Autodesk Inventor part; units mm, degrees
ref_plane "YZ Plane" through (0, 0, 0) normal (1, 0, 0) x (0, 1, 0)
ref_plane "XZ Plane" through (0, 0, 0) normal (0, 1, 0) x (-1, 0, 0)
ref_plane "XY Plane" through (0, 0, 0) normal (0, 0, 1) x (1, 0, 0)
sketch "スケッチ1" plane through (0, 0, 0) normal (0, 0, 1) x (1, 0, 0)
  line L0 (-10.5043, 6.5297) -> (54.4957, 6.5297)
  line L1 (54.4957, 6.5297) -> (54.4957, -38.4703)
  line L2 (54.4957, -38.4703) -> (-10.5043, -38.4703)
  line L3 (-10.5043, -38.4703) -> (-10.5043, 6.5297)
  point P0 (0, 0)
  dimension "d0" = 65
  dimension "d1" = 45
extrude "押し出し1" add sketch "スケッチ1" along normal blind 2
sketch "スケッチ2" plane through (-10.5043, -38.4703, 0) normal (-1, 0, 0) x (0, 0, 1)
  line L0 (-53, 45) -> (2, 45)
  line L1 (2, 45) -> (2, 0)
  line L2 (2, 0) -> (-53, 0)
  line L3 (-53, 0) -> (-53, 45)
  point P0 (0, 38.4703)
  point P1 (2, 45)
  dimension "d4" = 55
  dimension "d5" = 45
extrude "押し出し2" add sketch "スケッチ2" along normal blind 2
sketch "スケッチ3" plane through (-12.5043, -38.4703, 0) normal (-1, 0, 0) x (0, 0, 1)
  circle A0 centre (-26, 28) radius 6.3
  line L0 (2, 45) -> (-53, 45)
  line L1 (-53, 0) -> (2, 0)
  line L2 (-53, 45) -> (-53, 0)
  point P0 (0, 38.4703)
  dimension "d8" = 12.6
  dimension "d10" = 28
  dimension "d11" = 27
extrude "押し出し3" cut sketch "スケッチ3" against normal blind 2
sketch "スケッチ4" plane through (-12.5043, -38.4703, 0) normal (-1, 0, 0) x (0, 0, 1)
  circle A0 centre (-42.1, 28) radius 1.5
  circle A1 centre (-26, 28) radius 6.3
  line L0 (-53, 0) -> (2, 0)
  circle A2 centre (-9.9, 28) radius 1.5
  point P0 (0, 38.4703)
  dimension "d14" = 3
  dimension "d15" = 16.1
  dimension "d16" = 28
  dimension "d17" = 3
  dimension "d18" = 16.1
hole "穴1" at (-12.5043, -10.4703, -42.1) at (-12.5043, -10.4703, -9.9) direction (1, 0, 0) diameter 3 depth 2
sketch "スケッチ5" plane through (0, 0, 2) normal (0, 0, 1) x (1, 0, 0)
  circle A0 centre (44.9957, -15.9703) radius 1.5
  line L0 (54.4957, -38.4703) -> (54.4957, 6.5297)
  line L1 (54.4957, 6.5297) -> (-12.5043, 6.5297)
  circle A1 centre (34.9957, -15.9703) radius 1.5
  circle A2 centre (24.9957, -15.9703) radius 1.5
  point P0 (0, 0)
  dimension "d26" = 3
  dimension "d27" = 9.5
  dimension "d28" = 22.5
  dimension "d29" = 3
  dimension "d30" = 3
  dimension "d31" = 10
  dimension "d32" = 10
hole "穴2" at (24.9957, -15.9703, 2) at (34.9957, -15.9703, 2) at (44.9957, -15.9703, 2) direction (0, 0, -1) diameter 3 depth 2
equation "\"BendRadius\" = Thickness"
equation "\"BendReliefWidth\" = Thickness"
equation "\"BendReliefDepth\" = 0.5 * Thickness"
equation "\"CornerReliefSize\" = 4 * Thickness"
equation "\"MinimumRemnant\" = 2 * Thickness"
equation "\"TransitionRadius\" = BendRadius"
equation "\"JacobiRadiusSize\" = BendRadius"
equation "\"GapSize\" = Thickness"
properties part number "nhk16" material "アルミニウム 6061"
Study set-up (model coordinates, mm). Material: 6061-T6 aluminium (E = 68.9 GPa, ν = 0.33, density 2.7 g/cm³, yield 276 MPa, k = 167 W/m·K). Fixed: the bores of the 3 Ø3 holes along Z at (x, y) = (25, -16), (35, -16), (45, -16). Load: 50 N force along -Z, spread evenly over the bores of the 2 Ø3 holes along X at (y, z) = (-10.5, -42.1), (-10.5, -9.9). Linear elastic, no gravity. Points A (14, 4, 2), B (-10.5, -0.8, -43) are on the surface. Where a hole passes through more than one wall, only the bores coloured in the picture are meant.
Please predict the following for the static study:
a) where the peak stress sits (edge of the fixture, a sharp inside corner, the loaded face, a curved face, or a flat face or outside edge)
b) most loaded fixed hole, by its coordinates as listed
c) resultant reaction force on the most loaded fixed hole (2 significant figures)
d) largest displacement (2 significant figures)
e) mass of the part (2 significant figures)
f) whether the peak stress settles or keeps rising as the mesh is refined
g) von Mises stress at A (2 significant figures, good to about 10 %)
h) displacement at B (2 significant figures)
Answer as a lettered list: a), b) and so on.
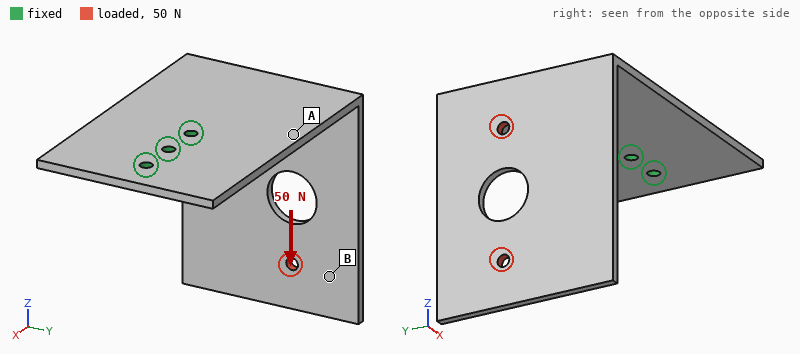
a) edge of the fixture
b) (25, -16)
c) 130 N
d) 1.1 mm
e) 28 g
f) keeps rising
g) 39 MPa
h) 0.90 mm
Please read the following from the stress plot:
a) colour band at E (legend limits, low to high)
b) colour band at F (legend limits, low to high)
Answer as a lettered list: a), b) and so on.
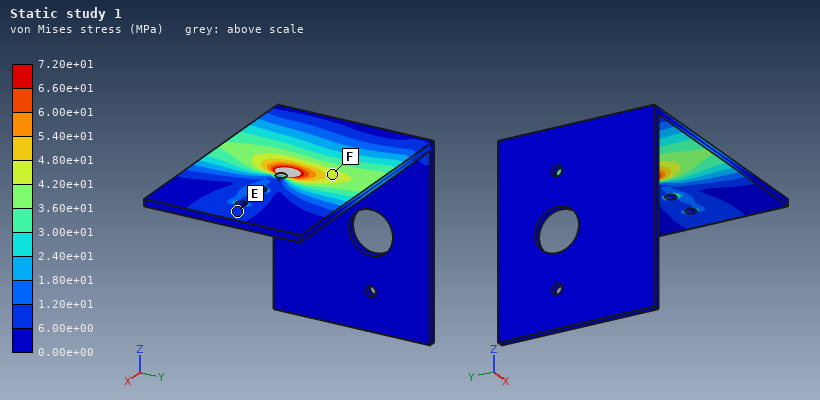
a) 6.00e+00 to 1.20e+01 MPa
b) 4.20e+01 to 4.80e+01 MPa
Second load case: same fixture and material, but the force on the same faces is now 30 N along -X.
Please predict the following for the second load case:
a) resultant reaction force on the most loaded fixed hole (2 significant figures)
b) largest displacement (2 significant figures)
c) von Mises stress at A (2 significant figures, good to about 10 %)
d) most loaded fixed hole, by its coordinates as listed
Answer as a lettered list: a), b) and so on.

a) 44 N
b) 1.1 mm
c) 25 MPa
d) (25, -16)
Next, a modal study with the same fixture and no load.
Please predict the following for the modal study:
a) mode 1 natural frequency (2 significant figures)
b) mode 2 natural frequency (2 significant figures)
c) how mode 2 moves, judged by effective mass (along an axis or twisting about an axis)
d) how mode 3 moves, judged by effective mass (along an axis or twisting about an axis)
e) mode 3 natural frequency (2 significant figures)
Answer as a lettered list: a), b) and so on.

a) 260 Hz
b) 390 Hz
c) along Y
d) along Z
e) 730 Hz
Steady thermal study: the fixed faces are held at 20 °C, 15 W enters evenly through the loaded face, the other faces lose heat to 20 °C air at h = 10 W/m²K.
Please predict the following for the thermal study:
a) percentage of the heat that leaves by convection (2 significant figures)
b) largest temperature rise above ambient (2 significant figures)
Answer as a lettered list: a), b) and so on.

a) 22 %
b) 67 K
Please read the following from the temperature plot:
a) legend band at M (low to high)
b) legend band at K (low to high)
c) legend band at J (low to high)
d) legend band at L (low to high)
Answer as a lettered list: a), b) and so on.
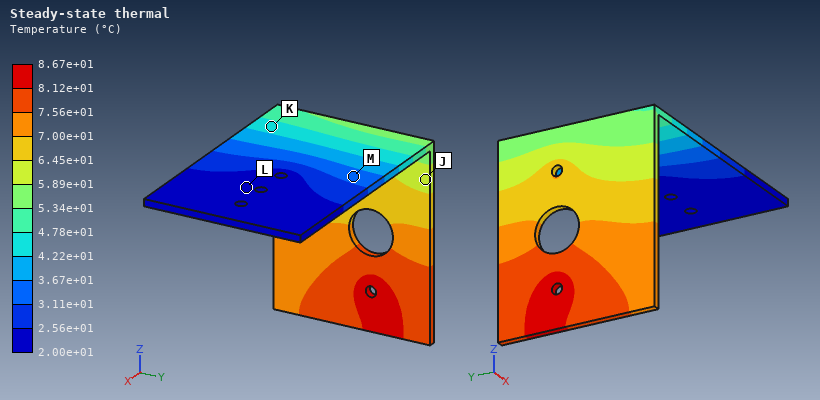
a) 3.11e+01 to 3.67e+01 °C
b) 4.22e+01 to 4.78e+01 °C
c) 5.89e+01 to 6.45e+01 °C
d) 2.00e+01 to 2.56e+01 °C
